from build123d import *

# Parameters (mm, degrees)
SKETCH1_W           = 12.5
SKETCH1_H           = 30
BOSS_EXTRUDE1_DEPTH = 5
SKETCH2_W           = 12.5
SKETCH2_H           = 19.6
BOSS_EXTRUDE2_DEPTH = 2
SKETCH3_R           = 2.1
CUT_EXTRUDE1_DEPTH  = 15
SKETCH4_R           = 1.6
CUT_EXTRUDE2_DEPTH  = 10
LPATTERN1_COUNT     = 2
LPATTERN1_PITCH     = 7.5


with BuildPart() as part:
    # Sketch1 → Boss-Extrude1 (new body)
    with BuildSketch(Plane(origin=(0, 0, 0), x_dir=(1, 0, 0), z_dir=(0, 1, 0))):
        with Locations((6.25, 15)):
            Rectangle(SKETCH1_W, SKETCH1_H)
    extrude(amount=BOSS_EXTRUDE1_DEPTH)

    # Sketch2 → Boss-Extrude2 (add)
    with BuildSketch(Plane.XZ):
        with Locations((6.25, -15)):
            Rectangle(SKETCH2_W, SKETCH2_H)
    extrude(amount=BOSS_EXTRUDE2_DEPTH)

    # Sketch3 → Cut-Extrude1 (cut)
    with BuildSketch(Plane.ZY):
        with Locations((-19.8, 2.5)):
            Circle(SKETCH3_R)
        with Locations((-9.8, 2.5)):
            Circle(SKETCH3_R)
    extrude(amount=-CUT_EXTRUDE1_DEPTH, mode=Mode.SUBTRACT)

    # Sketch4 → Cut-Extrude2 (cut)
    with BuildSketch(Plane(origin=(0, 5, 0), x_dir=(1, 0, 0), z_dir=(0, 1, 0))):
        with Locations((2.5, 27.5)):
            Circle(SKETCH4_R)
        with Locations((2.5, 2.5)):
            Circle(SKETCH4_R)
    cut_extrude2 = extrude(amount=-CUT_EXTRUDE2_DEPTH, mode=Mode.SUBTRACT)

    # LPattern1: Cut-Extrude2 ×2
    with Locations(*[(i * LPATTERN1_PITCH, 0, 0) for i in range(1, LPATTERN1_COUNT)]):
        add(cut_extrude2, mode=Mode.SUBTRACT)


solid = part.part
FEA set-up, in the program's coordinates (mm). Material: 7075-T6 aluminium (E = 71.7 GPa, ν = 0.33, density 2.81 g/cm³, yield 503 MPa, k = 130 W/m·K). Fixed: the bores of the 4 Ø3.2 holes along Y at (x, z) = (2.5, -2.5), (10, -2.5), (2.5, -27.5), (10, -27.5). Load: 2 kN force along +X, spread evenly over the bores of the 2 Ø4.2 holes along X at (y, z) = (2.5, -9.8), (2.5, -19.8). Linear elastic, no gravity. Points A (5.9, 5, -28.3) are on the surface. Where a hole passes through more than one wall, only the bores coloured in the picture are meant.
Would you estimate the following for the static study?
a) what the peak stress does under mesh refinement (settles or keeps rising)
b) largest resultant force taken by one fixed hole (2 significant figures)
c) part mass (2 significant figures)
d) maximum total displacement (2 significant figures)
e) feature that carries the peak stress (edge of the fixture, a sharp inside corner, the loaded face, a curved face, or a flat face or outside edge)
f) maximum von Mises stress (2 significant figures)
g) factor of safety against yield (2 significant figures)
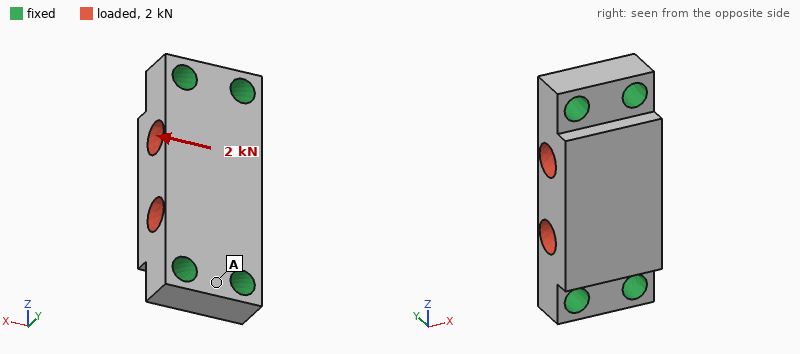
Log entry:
settles
700 N
5.2 g
9.9 µm
the loaded face
110 MPa
4.7
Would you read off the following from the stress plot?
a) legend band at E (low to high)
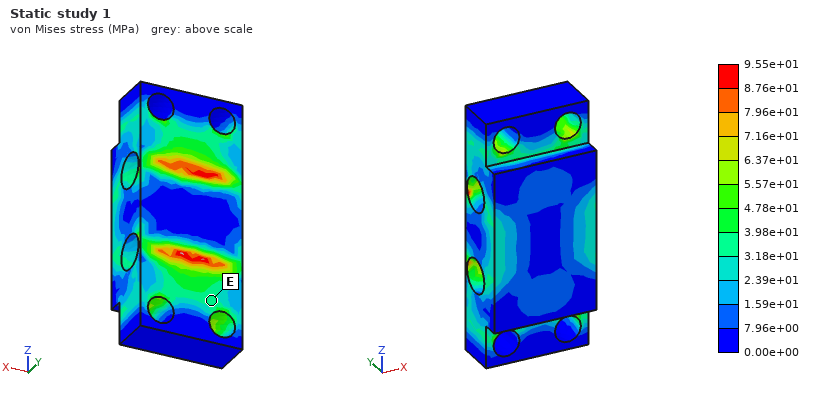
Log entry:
3.18e+01 to 3.98e+01 MPa
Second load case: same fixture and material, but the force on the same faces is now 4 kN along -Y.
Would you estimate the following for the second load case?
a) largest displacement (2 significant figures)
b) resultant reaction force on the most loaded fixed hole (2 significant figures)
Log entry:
30 µm
1.1 kN
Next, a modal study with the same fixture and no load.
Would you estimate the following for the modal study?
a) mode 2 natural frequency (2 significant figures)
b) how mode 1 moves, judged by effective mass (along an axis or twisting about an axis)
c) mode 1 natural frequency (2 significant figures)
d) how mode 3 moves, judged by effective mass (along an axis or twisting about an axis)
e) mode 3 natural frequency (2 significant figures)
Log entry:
45 kHz
along Y
33 kHz
along X
48 kHz
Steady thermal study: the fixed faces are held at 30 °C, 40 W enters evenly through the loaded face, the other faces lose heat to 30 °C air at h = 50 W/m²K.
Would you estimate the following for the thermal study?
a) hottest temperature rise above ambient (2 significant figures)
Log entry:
21 K
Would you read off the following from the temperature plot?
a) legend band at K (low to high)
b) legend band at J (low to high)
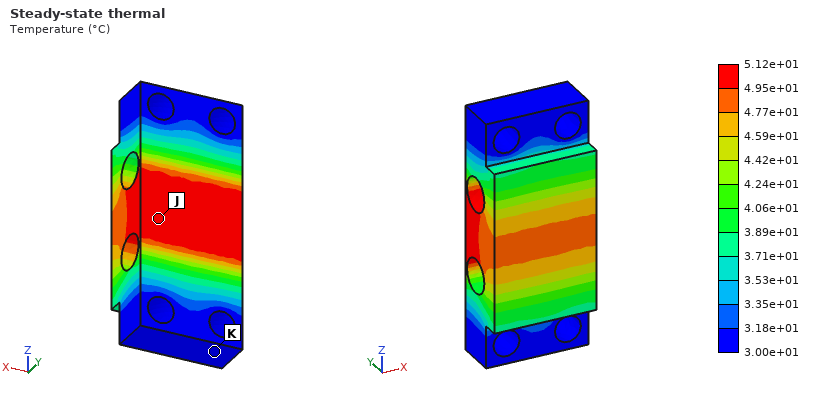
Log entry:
3.00e+01 to 3.18e+01 °C
4.95e+01 to 5.12e+01 °C
